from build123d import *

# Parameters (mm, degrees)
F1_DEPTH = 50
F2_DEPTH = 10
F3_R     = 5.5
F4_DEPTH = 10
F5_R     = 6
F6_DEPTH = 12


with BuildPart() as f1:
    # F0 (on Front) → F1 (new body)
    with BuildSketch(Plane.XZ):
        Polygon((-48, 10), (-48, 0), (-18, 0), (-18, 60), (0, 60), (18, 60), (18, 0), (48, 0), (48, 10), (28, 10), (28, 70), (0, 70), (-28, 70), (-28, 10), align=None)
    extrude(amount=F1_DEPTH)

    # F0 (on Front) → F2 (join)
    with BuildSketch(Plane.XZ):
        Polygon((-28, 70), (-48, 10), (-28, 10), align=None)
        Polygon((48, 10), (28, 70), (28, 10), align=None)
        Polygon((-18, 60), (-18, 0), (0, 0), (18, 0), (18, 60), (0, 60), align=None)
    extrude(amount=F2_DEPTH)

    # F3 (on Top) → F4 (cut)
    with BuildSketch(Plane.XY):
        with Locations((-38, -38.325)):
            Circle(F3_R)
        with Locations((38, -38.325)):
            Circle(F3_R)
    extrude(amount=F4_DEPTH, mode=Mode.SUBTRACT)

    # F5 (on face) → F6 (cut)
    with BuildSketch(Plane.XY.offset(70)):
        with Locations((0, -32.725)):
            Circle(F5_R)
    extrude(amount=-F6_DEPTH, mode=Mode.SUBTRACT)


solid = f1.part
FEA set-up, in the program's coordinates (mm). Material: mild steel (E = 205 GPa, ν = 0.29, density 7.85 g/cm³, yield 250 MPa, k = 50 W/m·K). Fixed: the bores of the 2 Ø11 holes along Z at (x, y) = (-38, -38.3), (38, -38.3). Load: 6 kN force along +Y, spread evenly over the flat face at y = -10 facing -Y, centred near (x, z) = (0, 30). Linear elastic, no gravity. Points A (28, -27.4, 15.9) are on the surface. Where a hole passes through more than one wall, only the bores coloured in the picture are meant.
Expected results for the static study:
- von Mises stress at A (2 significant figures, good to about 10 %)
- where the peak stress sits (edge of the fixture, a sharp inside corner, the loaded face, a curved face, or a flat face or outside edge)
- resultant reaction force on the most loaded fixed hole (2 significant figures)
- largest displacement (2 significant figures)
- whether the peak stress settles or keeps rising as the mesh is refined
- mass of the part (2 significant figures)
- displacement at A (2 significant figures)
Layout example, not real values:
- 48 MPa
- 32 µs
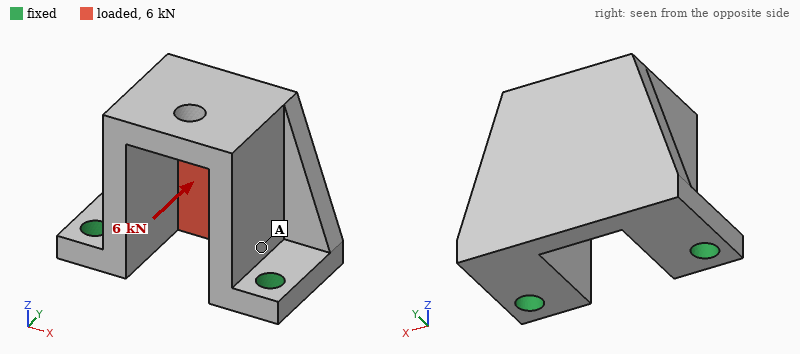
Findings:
- 22 MPa
- edge of the fixture
- 3.2 kN
- 67 µm
- keeps rising
- 1.1 kg
- 13 µm
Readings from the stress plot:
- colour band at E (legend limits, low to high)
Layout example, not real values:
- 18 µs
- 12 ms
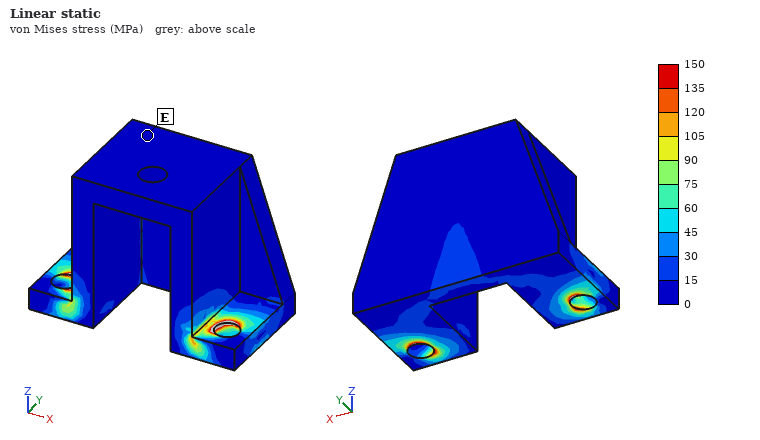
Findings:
- 0 to 15 MPa
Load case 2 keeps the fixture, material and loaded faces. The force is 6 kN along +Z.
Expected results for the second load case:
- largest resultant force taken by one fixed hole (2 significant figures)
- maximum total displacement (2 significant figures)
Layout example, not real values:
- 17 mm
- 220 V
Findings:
- 3.0 kN
- 68 µm
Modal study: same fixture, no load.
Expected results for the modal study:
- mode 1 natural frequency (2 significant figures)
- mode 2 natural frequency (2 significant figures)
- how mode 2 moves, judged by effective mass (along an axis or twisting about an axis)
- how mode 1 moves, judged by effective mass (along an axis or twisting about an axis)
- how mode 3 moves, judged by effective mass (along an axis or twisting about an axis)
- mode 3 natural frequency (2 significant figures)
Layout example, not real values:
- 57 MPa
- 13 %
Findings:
- 1500 Hz
- 2500 Hz
- along X
- along Y
- along X
- 5500 Hz
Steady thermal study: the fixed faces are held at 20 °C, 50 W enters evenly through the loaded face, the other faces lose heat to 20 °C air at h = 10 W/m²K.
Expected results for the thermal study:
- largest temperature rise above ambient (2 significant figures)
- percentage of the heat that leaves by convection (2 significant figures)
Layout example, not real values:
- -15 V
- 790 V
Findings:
- 44 K
- 16 %
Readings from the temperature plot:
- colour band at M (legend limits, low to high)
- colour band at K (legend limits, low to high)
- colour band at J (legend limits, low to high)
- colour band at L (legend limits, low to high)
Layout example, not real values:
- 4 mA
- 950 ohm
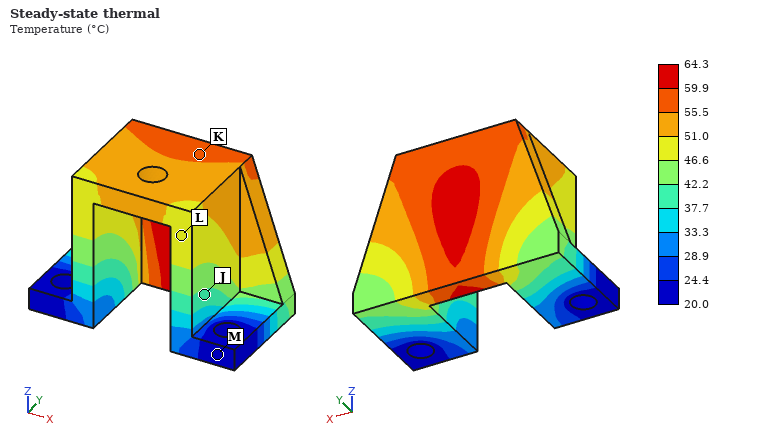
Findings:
- 20.0 to 24.4 °C
- 55.5 to 59.9 °C
- 37.7 to 42.2 °C
- 46.6 to 51.0 °C
